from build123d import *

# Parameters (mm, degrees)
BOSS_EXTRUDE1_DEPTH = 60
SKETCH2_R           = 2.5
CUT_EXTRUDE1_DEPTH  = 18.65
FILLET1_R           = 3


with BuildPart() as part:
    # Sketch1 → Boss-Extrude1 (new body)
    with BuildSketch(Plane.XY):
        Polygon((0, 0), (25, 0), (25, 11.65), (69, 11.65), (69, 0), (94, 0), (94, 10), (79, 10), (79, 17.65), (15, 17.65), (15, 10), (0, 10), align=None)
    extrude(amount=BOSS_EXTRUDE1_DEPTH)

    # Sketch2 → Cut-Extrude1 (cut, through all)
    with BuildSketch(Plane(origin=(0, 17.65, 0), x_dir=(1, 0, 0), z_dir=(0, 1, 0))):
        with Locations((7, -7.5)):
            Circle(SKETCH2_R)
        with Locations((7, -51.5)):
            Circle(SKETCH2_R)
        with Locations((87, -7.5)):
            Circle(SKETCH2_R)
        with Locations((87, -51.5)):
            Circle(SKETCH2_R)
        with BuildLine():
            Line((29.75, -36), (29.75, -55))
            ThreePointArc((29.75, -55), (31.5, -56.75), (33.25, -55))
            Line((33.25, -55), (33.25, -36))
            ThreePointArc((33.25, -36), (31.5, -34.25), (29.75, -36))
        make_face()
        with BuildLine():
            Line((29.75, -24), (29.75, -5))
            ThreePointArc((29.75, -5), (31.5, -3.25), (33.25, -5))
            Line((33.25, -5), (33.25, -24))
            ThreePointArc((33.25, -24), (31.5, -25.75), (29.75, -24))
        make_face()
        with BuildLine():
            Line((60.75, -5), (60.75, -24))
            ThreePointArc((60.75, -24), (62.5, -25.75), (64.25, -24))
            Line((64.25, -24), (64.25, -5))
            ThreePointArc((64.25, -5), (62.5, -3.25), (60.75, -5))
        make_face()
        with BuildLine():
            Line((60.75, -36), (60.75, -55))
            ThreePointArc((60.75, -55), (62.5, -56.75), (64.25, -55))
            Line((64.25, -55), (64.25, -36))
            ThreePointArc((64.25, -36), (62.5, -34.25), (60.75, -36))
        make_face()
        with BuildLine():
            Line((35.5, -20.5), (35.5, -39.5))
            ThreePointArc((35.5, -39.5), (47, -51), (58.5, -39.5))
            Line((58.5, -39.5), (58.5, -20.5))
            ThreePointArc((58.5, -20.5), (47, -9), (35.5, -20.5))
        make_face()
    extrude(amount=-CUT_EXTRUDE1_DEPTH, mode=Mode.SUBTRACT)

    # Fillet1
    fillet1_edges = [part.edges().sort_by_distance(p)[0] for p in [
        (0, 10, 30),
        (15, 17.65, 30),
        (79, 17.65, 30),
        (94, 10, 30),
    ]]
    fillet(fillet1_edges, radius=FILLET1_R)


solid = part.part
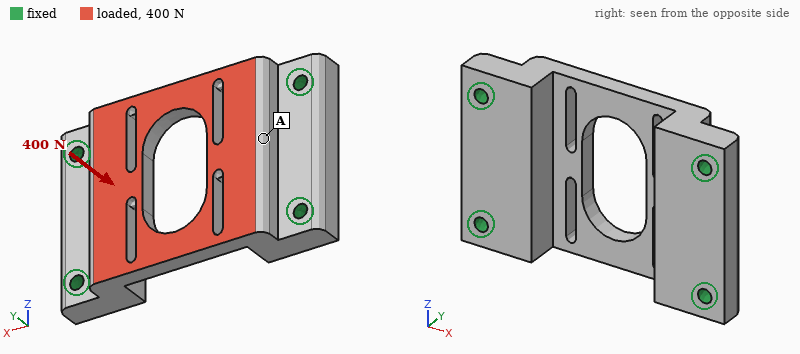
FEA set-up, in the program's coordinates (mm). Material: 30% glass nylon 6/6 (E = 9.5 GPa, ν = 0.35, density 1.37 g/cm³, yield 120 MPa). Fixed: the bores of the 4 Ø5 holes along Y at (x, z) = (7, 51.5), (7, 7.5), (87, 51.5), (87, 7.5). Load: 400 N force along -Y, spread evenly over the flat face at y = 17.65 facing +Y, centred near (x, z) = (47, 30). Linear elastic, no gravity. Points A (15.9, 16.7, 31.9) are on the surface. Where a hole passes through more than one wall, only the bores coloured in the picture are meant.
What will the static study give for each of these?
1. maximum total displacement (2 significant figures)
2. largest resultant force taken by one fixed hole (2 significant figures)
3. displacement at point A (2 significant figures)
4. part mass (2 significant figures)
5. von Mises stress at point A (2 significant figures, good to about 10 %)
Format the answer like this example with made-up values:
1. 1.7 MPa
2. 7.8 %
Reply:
1. 40 µm
2. 120 N
3. 12 µm
4. 64 g
5. 0.98 MPa
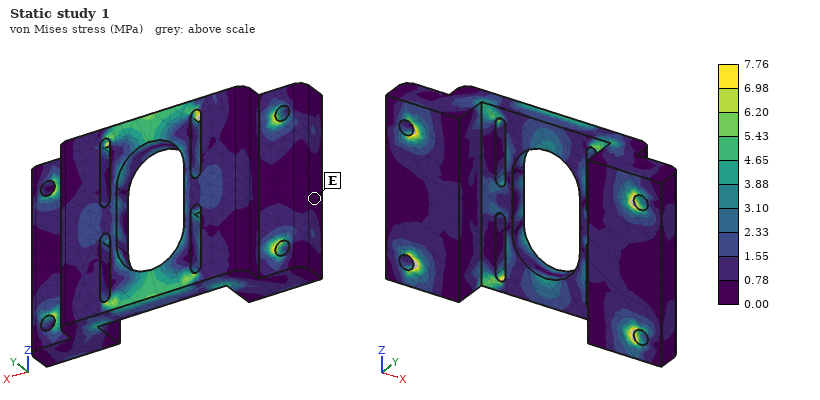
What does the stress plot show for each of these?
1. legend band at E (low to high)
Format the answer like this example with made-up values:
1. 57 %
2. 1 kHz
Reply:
1. 0.00 to 0.78 MPa
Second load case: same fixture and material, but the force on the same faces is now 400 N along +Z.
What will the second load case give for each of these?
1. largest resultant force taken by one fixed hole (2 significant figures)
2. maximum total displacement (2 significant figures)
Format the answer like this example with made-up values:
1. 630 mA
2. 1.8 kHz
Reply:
1. 140 N
2. 14 µm
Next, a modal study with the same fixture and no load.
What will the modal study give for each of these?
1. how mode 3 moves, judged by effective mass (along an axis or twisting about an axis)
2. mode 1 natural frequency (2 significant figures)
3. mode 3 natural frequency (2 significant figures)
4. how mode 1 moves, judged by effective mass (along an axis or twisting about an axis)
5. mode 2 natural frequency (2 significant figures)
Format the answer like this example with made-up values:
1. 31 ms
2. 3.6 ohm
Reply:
1. twisting about X
2. 4000 Hz
3. 4900 Hz
4. along Y
5. 4500 Hz
